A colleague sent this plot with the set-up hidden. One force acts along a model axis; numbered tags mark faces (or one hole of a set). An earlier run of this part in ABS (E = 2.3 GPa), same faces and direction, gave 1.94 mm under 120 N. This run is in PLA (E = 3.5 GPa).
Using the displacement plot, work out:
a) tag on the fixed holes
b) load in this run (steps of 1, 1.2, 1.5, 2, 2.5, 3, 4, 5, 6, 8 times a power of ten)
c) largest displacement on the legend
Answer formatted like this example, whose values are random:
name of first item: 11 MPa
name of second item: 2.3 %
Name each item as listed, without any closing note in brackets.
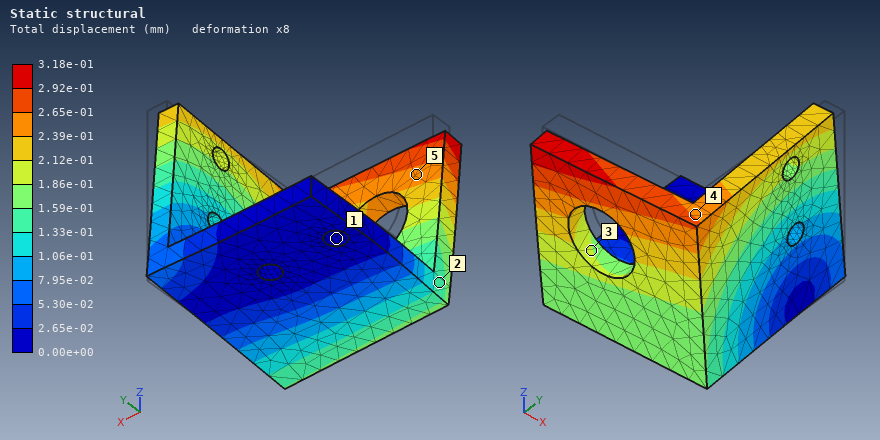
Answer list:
tag on the fixed holes: 1
load in this run: 30 N
largest displacement on the legend: 3.18e-01 mm
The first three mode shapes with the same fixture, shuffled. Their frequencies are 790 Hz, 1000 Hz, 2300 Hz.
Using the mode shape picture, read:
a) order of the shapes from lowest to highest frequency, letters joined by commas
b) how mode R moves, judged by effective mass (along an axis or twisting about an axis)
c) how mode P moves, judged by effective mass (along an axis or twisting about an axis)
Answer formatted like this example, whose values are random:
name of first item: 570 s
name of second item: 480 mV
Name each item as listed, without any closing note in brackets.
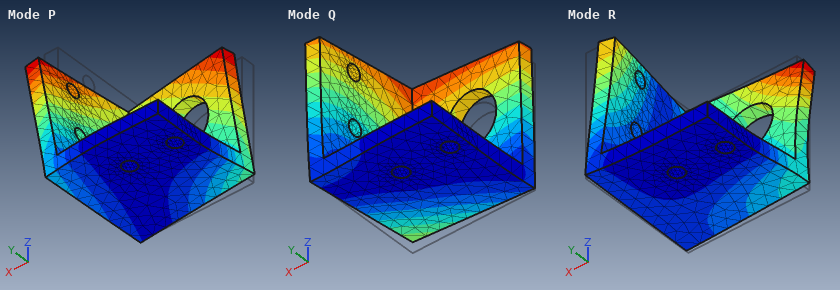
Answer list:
order of the shapes from lowest to highest frequency, letters joined by commas: Q, P, R
how mode R moves, judged by effective mass: along Z
how mode P moves, judged by effective mass: along X
